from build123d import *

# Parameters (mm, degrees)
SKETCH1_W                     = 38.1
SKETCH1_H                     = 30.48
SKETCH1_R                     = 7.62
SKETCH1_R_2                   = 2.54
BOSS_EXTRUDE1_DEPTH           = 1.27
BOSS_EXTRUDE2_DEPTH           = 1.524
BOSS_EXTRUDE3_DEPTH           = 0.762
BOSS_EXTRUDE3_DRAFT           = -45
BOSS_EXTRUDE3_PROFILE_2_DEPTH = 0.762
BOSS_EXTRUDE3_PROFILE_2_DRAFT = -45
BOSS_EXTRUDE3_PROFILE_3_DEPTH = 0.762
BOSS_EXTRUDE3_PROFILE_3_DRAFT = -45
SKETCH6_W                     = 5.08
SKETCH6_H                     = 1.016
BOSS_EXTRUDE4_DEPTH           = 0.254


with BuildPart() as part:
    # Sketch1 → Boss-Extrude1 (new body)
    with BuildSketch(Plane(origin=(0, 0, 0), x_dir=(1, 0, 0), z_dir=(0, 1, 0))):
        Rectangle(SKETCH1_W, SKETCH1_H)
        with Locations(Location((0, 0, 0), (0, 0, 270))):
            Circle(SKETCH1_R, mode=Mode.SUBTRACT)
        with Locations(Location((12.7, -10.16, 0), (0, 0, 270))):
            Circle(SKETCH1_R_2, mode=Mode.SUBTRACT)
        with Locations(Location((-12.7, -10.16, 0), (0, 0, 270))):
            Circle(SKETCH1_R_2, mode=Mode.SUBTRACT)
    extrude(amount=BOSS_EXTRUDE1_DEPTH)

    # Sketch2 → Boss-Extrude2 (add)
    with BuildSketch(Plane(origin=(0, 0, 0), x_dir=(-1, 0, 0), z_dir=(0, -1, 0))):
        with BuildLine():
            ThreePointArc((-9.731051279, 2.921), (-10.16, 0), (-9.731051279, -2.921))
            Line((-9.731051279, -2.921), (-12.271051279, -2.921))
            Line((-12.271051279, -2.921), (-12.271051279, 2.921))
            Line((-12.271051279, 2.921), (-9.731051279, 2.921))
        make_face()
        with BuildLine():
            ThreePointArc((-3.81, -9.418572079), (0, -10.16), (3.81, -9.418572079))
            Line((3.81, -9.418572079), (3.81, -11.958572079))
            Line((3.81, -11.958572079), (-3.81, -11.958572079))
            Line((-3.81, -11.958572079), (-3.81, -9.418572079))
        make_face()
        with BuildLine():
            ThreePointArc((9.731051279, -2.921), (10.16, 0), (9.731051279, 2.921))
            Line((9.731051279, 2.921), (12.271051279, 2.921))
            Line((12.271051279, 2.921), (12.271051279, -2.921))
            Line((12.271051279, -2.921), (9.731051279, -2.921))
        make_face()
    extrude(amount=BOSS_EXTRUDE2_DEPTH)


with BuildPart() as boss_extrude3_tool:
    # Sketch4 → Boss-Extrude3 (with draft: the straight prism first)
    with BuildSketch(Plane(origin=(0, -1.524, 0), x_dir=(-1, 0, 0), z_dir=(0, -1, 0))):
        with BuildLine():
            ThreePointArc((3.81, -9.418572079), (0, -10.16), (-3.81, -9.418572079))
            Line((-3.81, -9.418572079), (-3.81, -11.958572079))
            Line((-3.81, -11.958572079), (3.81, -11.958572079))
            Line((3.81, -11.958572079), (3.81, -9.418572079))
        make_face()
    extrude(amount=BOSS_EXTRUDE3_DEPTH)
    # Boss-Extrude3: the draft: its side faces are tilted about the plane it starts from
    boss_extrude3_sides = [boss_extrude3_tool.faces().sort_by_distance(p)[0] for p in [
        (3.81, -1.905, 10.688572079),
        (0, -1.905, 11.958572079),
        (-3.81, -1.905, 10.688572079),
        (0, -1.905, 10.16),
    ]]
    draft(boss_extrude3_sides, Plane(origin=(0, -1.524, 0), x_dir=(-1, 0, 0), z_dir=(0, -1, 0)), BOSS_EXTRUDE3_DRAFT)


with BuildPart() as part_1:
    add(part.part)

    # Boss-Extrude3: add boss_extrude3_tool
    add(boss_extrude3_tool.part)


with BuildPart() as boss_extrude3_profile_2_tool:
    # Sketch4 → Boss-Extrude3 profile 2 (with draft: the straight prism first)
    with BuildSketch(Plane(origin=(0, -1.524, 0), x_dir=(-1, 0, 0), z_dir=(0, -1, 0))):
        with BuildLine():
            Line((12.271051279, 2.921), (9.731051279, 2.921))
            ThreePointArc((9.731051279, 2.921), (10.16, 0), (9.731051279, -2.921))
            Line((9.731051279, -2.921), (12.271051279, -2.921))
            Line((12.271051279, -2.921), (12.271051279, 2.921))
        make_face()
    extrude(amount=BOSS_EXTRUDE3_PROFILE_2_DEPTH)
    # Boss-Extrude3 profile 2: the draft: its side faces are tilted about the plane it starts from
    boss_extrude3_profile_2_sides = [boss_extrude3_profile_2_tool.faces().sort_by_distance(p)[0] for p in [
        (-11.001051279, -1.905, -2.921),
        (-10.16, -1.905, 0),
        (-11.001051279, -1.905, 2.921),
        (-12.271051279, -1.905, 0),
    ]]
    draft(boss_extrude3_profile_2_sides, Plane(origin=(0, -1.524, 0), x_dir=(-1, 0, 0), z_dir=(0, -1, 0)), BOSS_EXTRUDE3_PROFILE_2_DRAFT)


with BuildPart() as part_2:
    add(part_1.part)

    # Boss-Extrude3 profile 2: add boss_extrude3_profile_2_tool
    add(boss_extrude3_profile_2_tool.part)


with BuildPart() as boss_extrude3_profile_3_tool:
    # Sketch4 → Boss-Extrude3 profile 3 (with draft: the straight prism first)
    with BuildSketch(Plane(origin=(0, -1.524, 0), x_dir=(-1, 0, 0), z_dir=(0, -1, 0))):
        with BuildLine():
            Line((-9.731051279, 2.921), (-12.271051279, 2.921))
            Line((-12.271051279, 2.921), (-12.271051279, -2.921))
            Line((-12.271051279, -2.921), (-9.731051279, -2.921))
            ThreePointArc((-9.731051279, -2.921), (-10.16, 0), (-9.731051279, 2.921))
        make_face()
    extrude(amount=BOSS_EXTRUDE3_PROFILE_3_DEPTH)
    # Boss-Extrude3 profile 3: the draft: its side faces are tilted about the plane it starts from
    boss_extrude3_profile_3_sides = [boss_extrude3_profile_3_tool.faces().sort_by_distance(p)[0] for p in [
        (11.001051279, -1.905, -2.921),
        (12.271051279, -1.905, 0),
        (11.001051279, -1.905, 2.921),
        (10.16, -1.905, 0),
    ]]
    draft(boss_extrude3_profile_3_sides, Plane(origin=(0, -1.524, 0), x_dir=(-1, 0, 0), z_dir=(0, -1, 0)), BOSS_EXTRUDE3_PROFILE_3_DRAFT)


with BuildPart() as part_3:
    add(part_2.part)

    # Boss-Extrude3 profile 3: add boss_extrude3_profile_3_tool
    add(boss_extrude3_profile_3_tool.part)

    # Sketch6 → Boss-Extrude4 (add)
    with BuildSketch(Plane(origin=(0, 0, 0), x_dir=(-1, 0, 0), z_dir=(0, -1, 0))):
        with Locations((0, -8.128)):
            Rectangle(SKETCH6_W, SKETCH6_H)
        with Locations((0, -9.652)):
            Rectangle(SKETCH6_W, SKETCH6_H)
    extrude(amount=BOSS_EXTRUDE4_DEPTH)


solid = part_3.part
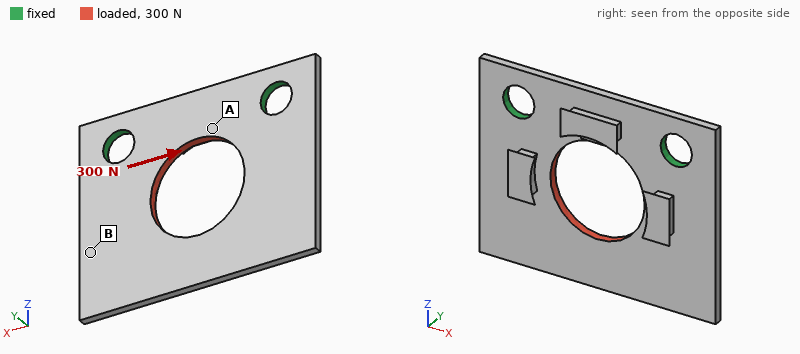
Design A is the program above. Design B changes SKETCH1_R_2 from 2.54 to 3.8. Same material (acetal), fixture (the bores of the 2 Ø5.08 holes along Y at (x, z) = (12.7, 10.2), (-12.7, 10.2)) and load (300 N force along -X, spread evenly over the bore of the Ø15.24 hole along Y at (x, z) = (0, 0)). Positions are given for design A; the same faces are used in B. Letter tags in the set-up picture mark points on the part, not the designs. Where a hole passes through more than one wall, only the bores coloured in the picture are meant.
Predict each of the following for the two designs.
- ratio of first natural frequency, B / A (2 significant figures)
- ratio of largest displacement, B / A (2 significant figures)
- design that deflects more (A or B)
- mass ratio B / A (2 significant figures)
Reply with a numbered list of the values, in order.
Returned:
1. 1.1
2. 0.80
3. A
4. 0.95
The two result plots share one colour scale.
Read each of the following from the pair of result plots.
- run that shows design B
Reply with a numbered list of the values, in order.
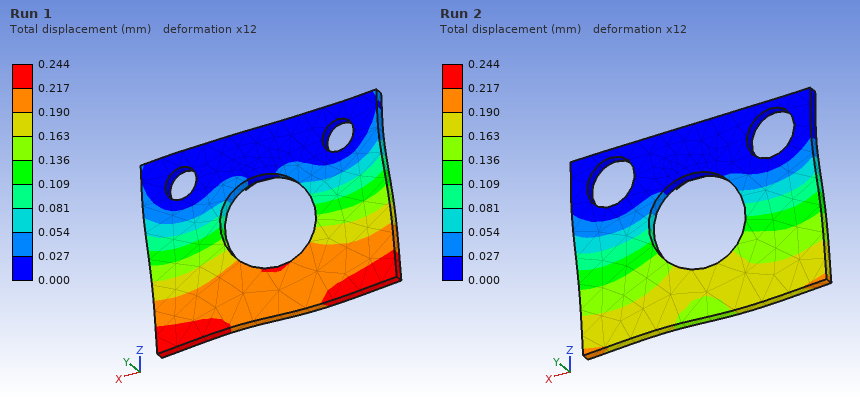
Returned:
1. Run 2
